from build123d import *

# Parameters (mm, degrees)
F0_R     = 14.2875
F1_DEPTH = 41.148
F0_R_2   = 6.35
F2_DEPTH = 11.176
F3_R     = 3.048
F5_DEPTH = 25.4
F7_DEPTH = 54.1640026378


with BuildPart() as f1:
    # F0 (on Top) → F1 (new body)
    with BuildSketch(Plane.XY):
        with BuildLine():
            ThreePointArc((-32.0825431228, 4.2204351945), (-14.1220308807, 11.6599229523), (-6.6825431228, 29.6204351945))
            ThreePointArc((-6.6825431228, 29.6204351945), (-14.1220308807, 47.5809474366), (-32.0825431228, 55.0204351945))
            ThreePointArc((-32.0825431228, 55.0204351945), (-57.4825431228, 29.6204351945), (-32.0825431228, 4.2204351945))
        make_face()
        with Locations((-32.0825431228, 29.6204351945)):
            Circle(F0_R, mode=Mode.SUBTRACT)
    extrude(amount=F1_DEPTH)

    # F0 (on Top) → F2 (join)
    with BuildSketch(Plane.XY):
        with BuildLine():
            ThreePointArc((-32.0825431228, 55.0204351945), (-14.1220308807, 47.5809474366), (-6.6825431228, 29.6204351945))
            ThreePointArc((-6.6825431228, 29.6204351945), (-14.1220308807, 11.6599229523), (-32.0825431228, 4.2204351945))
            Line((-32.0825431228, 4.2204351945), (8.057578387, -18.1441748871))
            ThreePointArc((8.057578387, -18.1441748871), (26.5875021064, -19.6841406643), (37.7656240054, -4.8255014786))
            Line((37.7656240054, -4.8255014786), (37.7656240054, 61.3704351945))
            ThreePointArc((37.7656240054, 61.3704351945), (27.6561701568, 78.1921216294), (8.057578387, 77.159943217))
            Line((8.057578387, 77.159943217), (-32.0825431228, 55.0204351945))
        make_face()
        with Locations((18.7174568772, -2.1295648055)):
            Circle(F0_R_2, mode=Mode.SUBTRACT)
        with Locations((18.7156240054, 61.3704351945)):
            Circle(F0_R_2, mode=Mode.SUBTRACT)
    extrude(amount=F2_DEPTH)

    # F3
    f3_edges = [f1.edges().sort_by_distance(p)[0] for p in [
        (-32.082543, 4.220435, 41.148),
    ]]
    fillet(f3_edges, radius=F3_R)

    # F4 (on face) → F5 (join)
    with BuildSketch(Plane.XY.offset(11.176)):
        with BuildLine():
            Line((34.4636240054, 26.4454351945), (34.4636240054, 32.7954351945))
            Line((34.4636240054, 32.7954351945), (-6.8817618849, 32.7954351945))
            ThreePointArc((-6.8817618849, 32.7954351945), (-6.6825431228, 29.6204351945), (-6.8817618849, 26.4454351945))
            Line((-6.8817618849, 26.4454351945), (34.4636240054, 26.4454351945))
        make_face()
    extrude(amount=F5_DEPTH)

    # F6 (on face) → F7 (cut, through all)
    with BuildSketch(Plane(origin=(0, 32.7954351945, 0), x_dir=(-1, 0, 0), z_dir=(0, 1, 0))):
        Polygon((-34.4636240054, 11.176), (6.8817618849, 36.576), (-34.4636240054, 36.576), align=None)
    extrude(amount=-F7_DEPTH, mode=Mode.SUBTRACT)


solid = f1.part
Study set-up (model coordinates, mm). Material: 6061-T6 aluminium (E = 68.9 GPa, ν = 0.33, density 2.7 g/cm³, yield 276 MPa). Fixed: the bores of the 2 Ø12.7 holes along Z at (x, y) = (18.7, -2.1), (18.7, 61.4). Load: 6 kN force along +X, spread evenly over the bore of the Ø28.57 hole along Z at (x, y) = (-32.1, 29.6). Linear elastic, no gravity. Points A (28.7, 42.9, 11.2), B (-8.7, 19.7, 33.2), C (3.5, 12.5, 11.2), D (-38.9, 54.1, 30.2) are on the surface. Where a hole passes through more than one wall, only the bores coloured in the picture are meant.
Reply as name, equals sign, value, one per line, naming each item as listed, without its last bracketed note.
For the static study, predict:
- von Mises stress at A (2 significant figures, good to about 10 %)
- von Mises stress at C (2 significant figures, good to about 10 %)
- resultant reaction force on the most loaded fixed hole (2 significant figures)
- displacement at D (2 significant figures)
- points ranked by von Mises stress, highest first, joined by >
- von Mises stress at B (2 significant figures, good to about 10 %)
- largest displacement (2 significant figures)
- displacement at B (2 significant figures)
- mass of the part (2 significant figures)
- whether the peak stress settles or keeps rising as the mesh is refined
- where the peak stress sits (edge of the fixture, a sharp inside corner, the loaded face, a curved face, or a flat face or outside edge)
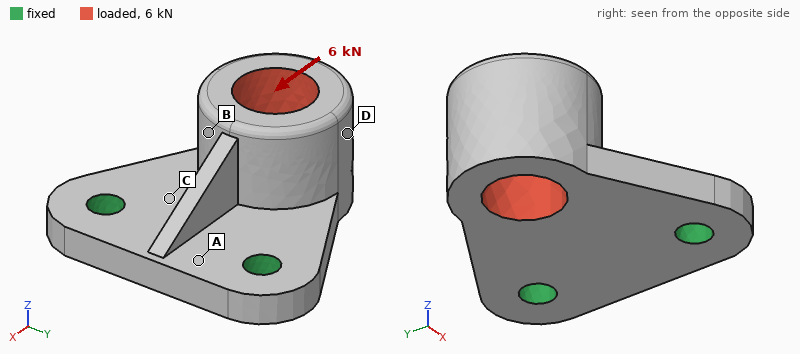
von Mises stress at A = 20 MPa
von Mises stress at C = 29 MPa
resultant reaction force on the most loaded fixed hole = 3.1 kN
displacement at D = 0.13 mm
points ranked by von Mises stress, highest first, joined by > = C > A > B > D
von Mises stress at B = 11 MPa
largest displacement = 0.18 mm
displacement at B = 0.079 mm
mass of the part = 300 g
whether the peak stress settles or keeps rising as the mesh is refined = keeps rising
where the peak stress sits = edge of the fixture
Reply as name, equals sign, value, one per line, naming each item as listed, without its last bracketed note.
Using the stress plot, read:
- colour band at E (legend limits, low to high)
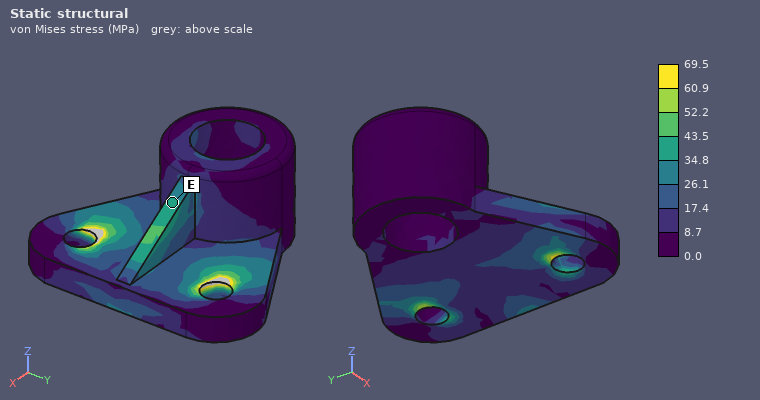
colour band at E = 34.8 to 43.5 MPa
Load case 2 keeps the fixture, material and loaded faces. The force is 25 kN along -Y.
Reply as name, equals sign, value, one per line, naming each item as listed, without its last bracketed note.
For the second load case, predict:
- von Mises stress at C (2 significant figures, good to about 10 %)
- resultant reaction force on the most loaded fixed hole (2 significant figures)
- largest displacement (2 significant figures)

von Mises stress at C = 110 MPa
resultant reaction force on the most loaded fixed hole = 23 kN
largest displacement = 0.31 mm
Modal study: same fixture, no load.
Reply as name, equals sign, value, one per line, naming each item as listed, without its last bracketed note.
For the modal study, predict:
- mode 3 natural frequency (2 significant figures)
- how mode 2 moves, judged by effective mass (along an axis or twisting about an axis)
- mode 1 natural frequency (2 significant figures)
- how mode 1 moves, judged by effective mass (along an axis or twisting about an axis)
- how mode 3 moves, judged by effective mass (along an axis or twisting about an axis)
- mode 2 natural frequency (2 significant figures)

mode 3 natural frequency = 6900 Hz
how mode 2 moves, judged by effective mass = along Y
mode 1 natural frequency = 1600 Hz
how mode 1 moves, judged by effective mass = along Z
how mode 3 moves, judged by effective mass = along Y
mode 2 natural frequency = 3900 Hz
